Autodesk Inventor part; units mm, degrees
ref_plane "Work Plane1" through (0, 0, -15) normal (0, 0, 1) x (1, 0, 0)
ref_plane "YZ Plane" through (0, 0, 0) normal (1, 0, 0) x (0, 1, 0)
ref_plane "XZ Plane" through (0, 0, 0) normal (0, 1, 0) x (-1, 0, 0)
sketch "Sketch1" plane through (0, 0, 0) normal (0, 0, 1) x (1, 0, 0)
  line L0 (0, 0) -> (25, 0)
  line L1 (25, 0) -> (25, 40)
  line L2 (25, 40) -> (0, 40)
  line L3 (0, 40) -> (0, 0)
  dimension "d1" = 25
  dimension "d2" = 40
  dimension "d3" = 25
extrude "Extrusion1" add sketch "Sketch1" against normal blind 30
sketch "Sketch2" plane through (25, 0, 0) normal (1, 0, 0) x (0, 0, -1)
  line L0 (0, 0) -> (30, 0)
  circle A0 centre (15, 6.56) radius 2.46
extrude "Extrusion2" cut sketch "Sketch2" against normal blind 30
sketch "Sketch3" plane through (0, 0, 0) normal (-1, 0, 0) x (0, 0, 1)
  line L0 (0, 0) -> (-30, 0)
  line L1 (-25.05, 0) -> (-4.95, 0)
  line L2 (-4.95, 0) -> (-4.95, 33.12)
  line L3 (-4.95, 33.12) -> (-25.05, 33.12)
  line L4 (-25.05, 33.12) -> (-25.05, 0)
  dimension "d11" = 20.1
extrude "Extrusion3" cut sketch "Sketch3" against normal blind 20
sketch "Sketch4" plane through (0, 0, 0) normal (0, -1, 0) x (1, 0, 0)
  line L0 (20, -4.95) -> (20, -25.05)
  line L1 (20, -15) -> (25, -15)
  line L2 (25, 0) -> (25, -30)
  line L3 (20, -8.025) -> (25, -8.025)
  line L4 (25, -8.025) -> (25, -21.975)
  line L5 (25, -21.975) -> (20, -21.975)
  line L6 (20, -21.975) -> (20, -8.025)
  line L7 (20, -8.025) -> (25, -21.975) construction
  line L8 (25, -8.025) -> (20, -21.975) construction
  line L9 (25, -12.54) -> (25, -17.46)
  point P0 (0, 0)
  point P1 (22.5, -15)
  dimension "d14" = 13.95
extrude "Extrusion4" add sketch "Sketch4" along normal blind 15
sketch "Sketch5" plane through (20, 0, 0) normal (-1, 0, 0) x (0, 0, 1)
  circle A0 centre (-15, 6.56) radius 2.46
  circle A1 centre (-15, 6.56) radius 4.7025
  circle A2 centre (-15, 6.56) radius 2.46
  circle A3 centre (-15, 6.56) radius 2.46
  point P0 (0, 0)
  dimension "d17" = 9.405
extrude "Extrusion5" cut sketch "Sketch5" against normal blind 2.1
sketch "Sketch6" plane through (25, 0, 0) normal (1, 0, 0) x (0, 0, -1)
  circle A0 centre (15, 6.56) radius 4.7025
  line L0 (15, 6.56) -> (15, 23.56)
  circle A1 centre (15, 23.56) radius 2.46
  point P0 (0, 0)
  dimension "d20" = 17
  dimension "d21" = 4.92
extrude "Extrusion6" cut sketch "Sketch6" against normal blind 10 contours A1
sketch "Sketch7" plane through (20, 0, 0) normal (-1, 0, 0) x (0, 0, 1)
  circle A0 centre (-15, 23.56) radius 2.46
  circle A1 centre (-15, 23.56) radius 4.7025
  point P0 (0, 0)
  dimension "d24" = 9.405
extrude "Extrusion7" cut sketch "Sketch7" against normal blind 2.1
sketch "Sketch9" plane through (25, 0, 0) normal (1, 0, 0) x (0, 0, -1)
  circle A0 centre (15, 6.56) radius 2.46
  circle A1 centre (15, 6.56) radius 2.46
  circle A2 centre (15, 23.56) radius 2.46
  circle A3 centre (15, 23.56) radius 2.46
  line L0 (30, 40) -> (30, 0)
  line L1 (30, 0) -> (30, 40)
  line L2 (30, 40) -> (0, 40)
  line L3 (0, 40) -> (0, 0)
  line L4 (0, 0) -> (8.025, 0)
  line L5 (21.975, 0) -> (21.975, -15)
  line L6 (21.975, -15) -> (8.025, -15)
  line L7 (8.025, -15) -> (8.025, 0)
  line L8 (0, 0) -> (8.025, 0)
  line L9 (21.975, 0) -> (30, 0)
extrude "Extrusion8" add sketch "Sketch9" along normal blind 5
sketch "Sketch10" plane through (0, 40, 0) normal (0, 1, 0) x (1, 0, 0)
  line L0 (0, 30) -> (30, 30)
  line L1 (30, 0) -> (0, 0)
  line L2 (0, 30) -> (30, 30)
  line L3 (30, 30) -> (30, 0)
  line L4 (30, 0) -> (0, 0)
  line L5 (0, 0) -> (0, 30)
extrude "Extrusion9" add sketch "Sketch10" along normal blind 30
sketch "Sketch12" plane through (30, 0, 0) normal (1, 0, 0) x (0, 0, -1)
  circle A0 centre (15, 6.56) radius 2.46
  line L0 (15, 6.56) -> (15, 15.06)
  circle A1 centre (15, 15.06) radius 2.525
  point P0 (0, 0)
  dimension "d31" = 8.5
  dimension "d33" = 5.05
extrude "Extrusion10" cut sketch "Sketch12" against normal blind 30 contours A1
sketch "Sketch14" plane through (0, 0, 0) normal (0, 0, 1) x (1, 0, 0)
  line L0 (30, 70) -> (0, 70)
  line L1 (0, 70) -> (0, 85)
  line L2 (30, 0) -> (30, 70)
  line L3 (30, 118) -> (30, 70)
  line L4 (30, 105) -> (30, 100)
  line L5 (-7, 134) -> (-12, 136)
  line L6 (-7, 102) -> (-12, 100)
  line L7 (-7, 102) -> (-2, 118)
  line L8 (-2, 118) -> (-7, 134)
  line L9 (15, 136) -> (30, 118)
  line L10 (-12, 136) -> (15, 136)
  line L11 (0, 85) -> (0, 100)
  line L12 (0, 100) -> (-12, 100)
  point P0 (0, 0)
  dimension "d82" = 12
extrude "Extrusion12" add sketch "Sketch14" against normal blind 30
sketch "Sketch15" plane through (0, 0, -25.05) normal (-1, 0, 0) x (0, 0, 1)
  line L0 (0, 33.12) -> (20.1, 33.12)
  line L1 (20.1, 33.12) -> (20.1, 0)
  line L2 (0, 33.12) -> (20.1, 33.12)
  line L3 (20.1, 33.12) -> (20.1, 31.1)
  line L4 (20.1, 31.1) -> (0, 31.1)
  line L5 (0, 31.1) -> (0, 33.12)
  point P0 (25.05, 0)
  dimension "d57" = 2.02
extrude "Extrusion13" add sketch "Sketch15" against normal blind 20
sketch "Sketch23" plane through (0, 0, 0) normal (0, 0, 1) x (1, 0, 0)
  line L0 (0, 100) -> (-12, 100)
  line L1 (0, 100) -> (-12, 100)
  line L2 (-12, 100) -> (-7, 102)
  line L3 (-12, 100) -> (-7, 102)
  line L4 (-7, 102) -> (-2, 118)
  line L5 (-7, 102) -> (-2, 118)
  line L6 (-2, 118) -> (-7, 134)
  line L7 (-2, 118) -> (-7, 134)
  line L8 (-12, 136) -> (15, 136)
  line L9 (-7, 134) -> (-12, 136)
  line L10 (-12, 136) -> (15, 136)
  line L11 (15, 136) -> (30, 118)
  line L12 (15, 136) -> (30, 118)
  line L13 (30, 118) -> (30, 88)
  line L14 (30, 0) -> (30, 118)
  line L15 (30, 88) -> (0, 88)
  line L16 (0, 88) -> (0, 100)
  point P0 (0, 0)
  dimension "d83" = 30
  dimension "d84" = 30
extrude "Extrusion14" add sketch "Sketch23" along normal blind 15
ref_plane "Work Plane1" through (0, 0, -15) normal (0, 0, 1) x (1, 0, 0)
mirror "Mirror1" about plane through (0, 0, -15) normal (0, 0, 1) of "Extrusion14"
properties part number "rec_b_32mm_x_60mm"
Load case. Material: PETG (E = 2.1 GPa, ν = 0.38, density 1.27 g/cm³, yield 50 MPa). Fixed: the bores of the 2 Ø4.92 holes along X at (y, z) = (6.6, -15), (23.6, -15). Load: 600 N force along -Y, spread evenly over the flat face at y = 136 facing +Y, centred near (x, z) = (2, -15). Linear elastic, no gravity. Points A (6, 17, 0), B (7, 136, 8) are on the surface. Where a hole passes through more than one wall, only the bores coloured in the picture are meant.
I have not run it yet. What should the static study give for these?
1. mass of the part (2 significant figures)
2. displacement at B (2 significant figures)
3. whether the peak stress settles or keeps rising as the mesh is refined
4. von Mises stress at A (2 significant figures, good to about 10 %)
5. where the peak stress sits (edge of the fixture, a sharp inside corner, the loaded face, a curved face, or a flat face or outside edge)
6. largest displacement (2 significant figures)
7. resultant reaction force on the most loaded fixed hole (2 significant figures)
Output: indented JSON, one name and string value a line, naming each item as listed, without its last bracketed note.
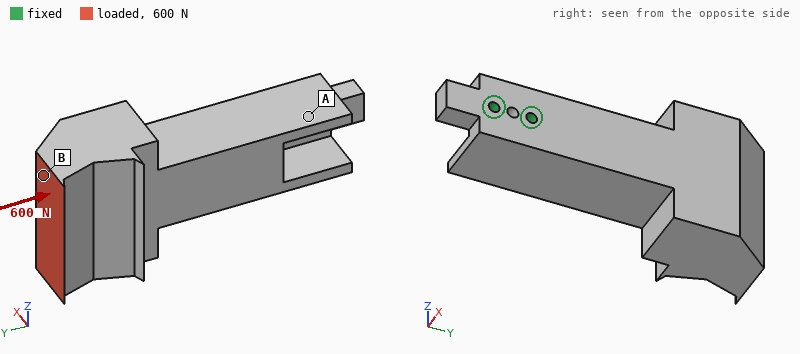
{
  "mass of the part": "200 g",
  "displacement at B": "1.5 mm",
  "whether the peak stress settles or keeps rising as the mesh is refined": "keeps rising",
  "von Mises stress at A": "3.2 MPa",
  "where the peak stress sits": "edge of the fixture",
  "largest displacement": "1.6 mm",
  "resultant reaction force on the most loaded fixed hole": "670 N"
}
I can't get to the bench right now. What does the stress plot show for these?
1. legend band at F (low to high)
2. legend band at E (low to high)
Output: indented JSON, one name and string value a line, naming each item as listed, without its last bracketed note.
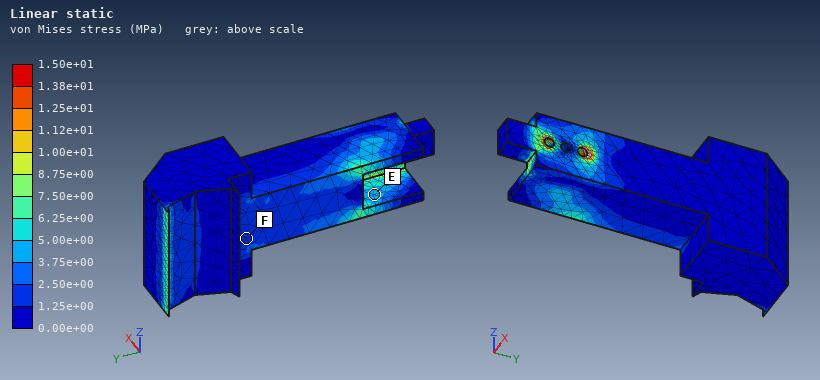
{
  "legend band at F": "1.25e+00 to 2.50e+00 MPa",
  "legend band at E": "3.75e+00 to 5.00e+00 MPa"
}
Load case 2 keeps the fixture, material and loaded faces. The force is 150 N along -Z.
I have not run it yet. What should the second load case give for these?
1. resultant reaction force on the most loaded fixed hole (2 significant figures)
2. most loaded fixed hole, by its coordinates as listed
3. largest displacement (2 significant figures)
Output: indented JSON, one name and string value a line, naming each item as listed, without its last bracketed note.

{
  "resultant reaction force on the most loaded fixed hole": "880 N",
  "most loaded fixed hole, by its coordinates as listed": "(23.6, -15)",
  "largest displacement": "1.5 mm"
}
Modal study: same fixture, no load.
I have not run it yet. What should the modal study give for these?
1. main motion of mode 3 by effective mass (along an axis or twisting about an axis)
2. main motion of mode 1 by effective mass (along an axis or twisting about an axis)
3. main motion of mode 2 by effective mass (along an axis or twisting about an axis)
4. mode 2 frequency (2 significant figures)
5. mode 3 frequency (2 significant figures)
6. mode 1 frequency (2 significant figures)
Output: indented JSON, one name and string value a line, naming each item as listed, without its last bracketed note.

{
  "main motion of mode 3 by effective mass": "twisting about Y",
  "main motion of mode 1 by effective mass": "along X",
  "main motion of mode 2 by effective mass": "along Z",
  "mode 2 frequency": "190 Hz",
  "mode 3 frequency": "460 Hz",
  "mode 1 frequency": "160 Hz"
}
